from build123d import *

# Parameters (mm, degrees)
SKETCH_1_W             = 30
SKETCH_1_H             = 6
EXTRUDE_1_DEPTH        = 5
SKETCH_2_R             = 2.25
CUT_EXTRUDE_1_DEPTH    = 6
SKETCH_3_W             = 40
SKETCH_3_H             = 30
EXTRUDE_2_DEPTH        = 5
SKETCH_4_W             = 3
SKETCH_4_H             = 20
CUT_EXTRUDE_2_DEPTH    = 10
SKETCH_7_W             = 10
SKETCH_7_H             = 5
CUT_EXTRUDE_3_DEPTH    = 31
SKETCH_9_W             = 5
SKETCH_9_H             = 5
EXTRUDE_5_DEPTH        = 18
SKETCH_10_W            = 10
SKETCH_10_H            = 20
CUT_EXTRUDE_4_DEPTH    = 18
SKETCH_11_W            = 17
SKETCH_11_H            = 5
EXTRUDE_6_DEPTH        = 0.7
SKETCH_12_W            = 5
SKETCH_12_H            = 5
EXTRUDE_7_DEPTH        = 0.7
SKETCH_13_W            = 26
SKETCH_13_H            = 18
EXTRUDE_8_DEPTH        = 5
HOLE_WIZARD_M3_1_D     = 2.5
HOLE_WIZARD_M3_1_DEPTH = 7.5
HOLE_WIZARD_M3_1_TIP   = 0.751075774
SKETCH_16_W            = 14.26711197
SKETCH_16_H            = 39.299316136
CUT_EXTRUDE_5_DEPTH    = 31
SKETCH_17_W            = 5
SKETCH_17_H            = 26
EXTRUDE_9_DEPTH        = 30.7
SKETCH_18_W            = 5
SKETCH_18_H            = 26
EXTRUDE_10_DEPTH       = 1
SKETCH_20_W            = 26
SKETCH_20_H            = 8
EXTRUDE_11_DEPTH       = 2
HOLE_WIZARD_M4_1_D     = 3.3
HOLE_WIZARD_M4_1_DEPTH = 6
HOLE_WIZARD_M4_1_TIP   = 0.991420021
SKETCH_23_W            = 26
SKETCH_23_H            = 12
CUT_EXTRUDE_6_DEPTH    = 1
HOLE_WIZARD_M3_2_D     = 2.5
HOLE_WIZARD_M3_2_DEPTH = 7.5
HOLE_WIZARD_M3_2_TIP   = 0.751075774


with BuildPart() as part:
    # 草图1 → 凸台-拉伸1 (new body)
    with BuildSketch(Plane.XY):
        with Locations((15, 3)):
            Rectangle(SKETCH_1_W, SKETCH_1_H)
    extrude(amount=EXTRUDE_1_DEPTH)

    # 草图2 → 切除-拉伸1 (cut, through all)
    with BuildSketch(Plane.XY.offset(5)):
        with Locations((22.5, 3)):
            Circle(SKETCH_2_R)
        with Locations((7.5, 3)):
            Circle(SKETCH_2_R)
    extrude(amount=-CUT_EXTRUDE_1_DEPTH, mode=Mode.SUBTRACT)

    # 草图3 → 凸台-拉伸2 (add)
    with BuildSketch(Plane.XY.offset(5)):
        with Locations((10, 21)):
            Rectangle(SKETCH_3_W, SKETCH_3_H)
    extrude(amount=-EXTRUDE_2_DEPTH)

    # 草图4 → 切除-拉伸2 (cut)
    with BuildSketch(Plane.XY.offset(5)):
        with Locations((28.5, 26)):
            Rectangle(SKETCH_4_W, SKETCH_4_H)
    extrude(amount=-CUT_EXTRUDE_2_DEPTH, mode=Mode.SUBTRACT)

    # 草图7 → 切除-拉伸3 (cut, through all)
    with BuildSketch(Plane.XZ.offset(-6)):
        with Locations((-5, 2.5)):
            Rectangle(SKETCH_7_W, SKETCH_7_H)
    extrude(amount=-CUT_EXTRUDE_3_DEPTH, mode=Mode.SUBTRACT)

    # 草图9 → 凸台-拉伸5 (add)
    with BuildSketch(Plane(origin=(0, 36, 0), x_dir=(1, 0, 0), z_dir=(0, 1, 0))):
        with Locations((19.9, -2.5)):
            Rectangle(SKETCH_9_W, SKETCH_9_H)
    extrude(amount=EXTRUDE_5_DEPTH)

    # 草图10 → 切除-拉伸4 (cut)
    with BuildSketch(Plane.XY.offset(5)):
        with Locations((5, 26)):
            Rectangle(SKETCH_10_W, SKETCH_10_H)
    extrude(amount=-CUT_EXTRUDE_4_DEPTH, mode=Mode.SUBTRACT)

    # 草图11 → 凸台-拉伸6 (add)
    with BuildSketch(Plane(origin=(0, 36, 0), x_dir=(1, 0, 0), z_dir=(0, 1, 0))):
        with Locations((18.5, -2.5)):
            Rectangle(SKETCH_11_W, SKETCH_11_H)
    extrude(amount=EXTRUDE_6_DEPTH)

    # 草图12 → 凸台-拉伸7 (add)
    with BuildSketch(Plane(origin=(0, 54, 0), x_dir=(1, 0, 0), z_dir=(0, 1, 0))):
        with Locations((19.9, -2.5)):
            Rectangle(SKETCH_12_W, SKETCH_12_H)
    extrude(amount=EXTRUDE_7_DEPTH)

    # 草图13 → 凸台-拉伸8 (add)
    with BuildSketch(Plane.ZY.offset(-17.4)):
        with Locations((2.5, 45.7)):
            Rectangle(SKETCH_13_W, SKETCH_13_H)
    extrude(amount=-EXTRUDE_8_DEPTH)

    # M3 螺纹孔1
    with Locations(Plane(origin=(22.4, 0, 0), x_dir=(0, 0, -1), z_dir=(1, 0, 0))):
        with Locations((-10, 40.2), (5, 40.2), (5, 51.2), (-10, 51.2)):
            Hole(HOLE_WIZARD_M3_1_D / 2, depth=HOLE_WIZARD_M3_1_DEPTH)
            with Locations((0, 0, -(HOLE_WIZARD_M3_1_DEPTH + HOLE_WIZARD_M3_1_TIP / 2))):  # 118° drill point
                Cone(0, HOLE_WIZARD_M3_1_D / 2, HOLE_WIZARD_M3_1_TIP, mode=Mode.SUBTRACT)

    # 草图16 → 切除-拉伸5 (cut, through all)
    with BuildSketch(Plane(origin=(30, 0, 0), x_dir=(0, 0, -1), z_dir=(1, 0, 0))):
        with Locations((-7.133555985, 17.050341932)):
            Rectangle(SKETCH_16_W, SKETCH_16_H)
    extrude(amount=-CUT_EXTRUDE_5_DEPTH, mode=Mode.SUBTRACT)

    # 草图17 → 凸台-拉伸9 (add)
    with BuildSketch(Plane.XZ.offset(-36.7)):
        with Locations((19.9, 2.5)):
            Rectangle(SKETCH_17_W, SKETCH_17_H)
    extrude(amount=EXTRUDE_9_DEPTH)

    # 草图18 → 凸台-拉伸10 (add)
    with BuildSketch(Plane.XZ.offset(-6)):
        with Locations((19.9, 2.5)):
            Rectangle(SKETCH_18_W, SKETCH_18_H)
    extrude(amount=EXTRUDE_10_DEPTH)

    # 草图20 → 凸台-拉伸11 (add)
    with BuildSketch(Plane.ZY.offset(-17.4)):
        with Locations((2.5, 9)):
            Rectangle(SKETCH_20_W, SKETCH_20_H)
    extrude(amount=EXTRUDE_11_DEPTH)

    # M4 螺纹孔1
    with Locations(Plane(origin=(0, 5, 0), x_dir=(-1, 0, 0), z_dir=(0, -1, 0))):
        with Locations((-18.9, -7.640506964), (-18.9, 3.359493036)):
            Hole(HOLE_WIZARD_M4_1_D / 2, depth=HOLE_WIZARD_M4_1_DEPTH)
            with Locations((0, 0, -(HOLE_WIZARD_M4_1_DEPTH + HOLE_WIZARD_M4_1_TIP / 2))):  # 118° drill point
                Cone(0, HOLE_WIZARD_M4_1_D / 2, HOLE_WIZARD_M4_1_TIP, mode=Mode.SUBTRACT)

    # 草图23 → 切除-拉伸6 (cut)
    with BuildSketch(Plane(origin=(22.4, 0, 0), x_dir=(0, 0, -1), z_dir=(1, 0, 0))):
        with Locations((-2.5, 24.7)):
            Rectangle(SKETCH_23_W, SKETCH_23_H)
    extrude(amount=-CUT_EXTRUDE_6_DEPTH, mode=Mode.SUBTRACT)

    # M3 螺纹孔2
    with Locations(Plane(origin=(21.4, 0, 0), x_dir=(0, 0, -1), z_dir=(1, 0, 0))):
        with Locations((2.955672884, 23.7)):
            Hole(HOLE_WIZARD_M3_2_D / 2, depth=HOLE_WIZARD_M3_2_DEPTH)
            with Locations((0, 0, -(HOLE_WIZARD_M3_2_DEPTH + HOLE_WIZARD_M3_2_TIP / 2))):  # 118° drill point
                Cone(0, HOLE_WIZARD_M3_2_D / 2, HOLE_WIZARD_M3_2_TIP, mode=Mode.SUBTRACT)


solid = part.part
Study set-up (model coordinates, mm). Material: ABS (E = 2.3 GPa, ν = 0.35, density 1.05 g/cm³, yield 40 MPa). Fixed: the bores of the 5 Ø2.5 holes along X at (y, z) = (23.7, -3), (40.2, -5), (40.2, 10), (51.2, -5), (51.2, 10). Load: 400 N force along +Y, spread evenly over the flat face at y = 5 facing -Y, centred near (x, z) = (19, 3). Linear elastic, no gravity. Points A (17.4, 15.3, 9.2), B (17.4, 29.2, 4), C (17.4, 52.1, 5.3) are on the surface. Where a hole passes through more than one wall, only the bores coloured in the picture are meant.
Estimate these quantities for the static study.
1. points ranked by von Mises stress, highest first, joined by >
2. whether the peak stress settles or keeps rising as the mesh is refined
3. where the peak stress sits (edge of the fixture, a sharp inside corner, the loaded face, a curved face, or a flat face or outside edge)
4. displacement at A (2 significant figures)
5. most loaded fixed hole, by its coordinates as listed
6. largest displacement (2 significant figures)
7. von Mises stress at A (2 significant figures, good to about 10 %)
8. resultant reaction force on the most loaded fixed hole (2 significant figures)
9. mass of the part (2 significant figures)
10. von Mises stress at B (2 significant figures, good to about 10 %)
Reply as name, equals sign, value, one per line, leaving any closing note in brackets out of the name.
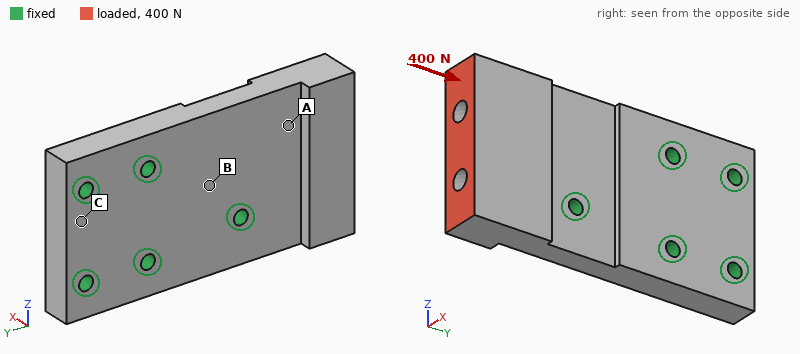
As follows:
points ranked by von Mises stress, highest first, joined by > = A > B > C
whether the peak stress settles or keeps rising as the mesh is refined = keeps rising
where the peak stress sits = edge of the fixture
displacement at A = 0.069 mm
most loaded fixed hole, by its coordinates as listed = (23.7, -3)
largest displacement = 0.17 mm
von Mises stress at A = 6.0 MPa
resultant reaction force on the most loaded fixed hole = 210 N
mass of the part = 6.7 g
von Mises stress at B = 3.2 MPa
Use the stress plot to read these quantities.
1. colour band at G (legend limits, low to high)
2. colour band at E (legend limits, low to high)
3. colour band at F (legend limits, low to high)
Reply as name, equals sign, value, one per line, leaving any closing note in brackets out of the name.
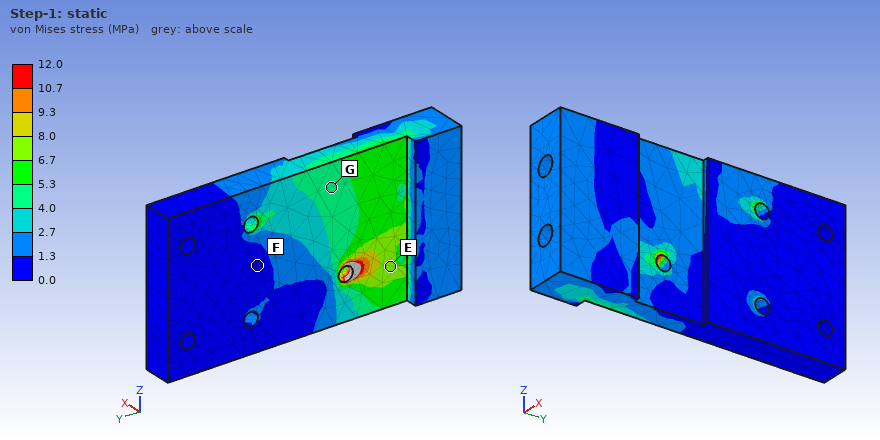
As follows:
colour band at G = 4.0 to 5.3 MPa
colour band at E = 6.7 to 8.0 MPa
colour band at F = 0.0 to 1.3 MPa
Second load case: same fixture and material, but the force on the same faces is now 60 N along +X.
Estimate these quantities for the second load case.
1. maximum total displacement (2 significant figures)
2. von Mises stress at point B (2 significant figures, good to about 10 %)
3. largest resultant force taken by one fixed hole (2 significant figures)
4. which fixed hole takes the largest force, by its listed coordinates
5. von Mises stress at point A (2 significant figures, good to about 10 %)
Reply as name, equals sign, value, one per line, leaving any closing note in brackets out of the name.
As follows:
maximum total displacement = 0.63 mm
von Mises stress at point B = 5.4 MPa
largest resultant force taken by one fixed hole = 91 N
which fixed hole takes the largest force, by its listed coordinates = (23.7, -3)
von Mises stress at point A = 4.8 MPa
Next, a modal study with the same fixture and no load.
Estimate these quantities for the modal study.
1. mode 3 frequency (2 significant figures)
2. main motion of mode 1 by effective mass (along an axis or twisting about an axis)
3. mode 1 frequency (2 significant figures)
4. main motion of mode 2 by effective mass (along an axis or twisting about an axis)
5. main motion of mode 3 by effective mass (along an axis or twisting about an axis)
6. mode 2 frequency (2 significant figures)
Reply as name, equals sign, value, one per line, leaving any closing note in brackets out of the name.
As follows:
mode 3 frequency = 5200 Hz
main motion of mode 1 by effective mass = along X
mode 1 frequency = 1600 Hz
main motion of mode 2 by effective mass = twisting about Y
main motion of mode 3 by effective mass = along Z
mode 2 frequency = 3200 Hz
